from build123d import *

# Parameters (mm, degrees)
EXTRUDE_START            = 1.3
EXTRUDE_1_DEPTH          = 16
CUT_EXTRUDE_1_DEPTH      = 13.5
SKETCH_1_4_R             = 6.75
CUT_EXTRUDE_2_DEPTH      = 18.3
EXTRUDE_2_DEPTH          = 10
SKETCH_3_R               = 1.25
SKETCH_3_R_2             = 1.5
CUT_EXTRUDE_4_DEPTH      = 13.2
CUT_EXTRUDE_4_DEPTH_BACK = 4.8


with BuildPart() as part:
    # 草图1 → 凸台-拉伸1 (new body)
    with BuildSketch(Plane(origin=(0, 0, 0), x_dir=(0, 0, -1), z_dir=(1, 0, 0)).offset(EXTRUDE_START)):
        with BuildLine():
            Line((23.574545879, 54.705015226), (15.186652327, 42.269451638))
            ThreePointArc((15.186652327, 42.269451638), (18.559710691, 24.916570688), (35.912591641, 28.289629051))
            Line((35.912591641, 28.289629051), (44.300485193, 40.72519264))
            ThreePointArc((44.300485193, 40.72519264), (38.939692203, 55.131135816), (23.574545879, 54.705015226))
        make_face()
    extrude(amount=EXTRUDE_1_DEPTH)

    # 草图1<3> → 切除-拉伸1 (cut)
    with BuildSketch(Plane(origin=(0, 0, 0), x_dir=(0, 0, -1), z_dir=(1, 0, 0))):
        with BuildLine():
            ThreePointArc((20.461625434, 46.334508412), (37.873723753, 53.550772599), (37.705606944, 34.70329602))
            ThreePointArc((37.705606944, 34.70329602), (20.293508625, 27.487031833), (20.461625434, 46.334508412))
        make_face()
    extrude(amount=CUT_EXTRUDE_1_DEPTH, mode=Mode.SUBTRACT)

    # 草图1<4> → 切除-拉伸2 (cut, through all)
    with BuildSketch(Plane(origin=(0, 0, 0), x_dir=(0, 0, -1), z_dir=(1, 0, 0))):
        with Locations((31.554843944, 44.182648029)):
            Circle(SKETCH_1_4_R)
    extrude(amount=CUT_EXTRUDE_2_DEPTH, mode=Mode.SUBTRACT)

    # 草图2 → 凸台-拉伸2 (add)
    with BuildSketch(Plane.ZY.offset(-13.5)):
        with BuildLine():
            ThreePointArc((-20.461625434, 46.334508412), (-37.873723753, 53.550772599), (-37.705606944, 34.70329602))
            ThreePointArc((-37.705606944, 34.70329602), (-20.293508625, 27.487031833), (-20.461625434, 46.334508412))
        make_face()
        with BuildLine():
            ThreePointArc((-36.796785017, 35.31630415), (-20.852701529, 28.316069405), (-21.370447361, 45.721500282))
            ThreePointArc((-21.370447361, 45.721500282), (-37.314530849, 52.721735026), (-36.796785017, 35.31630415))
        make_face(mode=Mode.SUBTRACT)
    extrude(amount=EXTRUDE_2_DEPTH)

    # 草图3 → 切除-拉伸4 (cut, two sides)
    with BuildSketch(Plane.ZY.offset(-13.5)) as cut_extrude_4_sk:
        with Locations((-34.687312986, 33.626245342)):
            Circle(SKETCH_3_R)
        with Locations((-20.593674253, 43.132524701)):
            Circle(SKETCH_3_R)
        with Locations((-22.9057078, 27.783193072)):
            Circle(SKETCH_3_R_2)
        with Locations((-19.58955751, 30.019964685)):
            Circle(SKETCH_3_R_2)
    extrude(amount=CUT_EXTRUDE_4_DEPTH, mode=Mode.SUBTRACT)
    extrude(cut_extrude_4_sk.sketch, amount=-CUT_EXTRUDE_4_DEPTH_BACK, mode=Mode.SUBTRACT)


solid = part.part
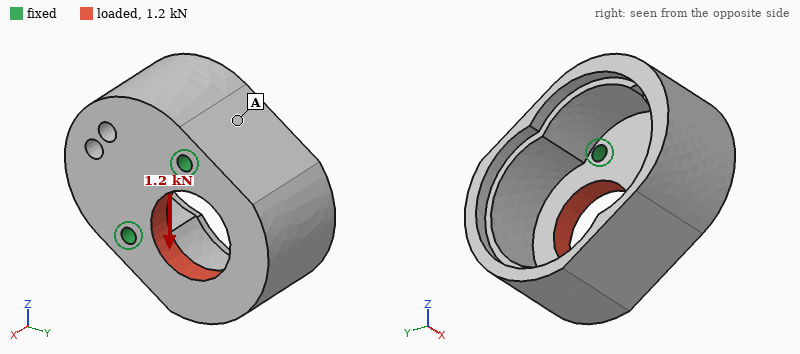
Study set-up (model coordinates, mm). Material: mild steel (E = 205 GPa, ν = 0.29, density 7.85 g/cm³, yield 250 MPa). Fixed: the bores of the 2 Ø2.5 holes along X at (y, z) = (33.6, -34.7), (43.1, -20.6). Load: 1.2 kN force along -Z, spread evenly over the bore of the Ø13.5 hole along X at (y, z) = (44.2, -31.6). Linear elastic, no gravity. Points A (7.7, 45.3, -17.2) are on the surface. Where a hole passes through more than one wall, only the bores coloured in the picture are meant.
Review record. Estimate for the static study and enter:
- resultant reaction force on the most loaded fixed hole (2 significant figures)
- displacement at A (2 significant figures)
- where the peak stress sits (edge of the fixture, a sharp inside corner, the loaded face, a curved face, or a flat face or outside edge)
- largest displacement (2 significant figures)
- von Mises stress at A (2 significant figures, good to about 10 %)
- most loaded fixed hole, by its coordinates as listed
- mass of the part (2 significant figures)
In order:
820 N
1.4 µm
edge of the fixture
5.8 µm
12 MPa
(43.1, -20.6)
43 g
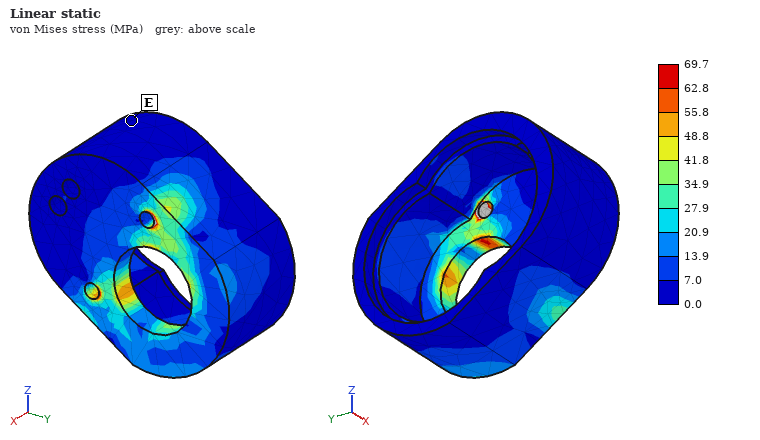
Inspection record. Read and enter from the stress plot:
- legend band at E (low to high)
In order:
0.0 to 7.0 MPa
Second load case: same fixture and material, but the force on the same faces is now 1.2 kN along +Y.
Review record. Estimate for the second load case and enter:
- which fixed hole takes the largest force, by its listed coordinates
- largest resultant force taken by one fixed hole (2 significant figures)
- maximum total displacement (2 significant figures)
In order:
(33.6, -34.7)
800 N
4.2 µm
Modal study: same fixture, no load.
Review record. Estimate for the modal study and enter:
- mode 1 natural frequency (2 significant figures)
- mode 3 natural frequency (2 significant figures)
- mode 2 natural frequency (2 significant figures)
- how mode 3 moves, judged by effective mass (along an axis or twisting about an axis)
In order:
6000 Hz
14 kHz
10 kHz
along X
